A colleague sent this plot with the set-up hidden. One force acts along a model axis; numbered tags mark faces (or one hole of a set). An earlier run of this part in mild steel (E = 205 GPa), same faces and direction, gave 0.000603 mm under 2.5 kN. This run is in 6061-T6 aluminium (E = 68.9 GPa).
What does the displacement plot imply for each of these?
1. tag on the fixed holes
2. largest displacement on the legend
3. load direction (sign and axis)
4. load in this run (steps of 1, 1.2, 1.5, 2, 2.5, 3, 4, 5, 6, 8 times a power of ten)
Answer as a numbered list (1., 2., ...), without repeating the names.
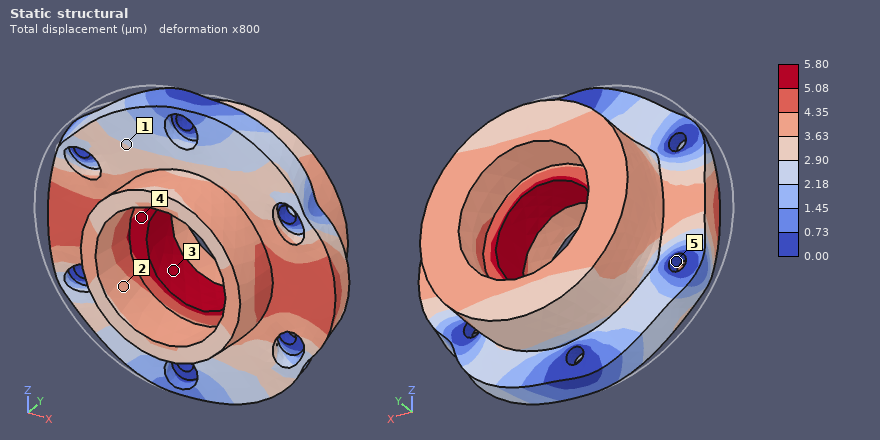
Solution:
1. 5
2. 5.80 µm
3. +X
4. 8 kN
